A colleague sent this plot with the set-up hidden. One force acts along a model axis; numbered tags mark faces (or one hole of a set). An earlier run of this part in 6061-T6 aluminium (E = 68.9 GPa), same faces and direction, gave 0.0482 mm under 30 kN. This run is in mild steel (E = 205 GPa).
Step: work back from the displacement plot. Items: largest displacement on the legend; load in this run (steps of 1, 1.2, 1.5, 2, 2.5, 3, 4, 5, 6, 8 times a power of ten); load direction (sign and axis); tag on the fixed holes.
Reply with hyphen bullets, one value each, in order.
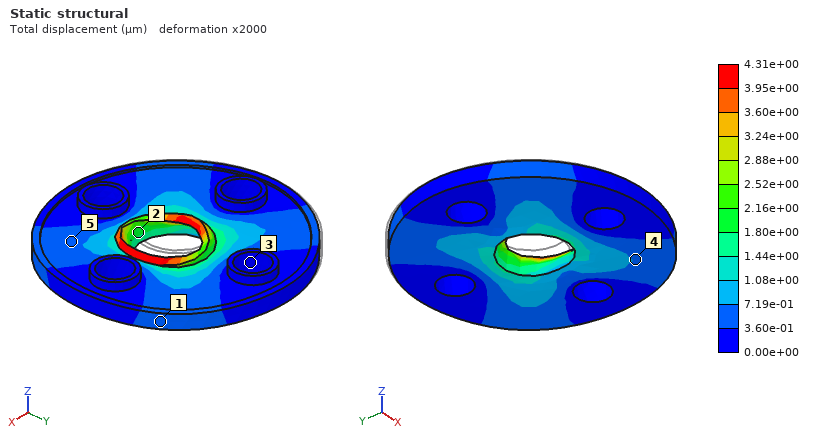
- 4.31e+00 µm
- 8 kN
- +X
- 3
